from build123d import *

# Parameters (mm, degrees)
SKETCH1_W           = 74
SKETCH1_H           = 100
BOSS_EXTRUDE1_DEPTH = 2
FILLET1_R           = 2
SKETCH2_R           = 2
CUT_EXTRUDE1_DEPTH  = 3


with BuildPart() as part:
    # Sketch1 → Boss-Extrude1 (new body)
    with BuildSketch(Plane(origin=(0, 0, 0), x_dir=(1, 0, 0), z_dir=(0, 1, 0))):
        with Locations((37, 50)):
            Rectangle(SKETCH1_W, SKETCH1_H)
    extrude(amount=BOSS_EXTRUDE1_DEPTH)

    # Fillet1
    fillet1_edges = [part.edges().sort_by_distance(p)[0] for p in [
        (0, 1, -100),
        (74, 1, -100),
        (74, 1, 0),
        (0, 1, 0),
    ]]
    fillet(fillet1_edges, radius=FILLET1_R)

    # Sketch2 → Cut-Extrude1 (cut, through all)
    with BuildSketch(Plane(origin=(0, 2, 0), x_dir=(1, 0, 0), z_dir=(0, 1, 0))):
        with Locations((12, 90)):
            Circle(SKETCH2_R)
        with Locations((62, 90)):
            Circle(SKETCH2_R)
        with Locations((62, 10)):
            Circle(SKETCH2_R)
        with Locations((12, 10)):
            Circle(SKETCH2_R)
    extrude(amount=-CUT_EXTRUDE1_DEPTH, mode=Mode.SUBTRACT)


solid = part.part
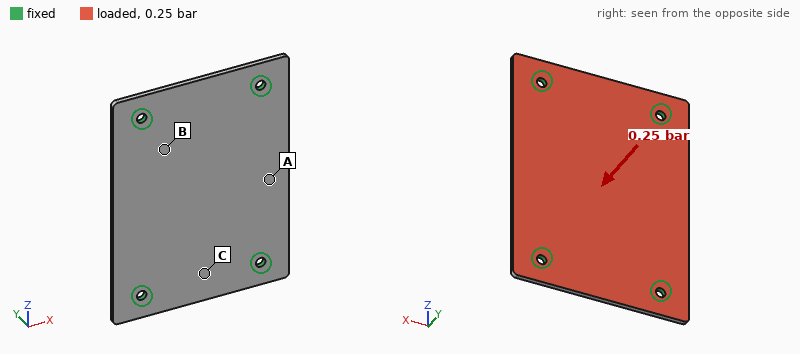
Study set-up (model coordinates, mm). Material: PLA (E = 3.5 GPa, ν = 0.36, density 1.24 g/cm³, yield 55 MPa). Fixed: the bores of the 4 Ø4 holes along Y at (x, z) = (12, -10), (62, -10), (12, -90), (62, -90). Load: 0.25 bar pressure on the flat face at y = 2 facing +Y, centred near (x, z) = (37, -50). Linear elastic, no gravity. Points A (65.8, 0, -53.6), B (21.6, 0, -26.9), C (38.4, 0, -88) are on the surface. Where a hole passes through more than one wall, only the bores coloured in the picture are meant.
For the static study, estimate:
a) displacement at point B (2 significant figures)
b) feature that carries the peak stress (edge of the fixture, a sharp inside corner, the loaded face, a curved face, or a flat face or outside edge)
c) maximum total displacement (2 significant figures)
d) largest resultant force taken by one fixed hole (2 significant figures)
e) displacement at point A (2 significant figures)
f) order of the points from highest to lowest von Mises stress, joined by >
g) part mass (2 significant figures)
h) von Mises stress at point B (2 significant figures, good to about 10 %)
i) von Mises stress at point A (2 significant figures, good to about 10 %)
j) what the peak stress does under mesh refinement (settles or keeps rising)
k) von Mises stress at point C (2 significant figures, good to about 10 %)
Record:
0.71 mm
edge of the fixture
1.4 mm
46 N
1.3 mm
A > C > B
18 g
3.0 MPa
10 MPa
keeps rising
5.9 MPa
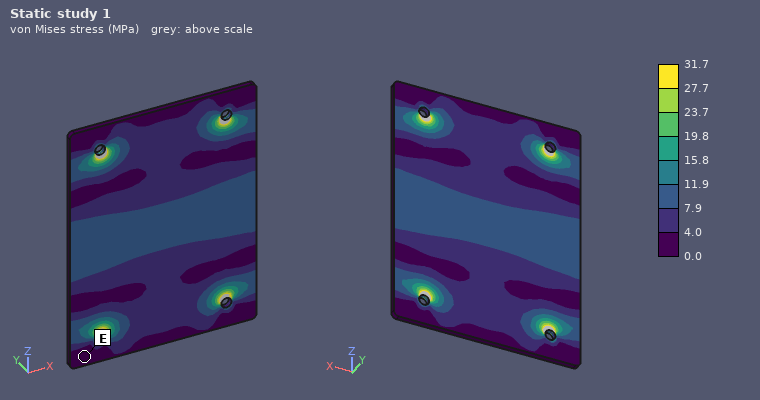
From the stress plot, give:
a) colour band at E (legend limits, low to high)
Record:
0.0 to 4.0 MPa
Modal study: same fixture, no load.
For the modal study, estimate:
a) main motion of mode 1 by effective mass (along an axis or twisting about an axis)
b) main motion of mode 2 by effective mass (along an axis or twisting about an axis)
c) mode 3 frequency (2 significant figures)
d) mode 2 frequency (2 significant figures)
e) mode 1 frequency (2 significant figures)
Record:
along Y
twisting about Z
1000 Hz
660 Hz
500 Hz
